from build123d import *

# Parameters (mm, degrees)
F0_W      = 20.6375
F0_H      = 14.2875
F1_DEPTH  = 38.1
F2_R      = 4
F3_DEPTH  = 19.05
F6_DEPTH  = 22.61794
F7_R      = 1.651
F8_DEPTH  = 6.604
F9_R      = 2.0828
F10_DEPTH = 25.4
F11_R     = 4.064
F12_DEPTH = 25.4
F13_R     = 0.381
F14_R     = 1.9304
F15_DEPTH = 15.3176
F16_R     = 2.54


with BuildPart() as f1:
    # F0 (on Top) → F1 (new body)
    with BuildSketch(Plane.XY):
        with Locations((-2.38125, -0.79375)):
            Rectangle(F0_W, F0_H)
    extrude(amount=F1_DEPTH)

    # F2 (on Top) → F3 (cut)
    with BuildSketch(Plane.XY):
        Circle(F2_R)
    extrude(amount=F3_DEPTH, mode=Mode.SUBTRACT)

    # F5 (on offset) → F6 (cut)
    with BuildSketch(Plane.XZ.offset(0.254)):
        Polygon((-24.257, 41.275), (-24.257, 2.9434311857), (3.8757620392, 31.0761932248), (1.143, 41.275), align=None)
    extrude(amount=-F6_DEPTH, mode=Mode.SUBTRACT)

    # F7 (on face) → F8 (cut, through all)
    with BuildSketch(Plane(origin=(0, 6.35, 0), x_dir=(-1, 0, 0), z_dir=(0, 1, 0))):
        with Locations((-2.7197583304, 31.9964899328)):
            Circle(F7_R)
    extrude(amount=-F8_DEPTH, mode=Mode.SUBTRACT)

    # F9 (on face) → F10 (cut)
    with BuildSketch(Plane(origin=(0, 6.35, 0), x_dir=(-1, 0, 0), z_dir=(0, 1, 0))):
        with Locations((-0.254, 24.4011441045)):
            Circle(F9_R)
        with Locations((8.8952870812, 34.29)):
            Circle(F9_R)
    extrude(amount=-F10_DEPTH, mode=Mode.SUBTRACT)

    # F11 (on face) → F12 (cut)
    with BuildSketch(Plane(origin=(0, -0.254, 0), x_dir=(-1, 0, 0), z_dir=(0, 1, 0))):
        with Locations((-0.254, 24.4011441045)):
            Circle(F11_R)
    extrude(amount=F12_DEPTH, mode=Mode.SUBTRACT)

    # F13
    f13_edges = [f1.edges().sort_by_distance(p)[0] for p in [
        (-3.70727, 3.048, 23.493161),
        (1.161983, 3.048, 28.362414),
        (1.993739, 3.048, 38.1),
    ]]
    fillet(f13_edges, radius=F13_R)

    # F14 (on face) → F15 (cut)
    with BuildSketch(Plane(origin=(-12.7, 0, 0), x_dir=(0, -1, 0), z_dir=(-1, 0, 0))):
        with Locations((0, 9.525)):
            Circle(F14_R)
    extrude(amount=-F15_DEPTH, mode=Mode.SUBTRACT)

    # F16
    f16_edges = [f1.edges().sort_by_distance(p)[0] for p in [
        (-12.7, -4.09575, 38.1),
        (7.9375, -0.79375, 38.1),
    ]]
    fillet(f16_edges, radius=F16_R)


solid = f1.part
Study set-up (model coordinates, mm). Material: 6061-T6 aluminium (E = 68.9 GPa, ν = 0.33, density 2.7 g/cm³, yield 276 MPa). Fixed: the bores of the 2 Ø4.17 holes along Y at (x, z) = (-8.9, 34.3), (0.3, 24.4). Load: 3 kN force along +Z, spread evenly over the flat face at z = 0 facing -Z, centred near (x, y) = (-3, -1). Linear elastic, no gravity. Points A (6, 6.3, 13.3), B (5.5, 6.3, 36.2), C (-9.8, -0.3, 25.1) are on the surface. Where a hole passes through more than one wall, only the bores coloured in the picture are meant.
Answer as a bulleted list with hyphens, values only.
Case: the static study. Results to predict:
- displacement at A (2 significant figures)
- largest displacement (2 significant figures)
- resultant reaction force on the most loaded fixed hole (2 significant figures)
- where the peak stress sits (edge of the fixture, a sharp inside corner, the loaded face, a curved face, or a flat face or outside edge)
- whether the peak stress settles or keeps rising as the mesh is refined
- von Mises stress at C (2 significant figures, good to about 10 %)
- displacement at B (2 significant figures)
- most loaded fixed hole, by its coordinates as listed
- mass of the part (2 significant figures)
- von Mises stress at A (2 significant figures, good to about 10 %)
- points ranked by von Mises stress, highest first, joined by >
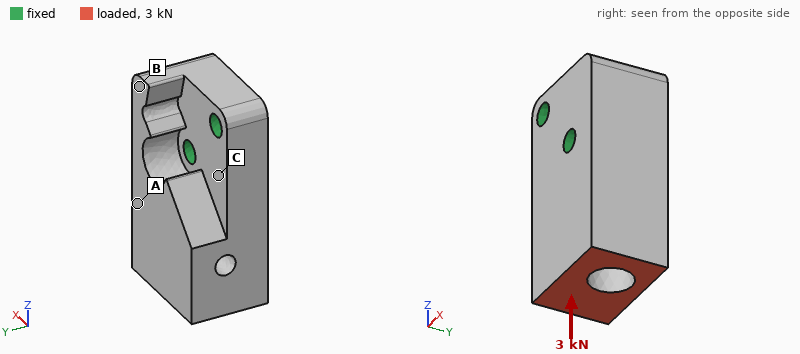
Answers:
- 15 µm
- 32 µm
- 2.0 kN
- a sharp inside corner
- keeps rising
- 36 MPa
- 8.4 µm
- (0.3, 24.4)
- 22 g
- 18 MPa
- C > A > B
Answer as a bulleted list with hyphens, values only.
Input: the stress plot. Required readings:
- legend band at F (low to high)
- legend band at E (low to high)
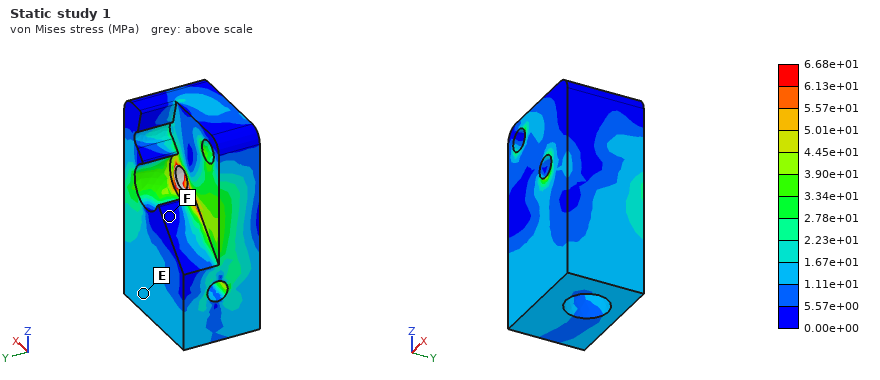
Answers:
- 0.00e+00 to 5.57e+00 MPa
- 1.11e+01 to 1.67e+01 MPa
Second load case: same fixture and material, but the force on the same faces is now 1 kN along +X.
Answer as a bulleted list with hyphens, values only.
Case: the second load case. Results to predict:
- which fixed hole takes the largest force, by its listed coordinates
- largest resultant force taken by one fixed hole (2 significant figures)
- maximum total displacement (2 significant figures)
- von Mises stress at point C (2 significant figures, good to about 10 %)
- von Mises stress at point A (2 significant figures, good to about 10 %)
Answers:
- (0.3, 24.4)
- 2.1 kN
- 34 µm
- 31 MPa
- 7.5 MPa
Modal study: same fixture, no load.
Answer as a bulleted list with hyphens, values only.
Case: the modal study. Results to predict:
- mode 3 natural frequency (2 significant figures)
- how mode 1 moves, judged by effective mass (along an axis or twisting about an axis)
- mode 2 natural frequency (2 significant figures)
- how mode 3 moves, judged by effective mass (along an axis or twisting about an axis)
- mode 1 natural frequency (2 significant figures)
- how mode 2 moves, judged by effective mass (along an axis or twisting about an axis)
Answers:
- 17 kHz
- along Y
- 12 kHz
- twisting about Z
- 8400 Hz
- along X
